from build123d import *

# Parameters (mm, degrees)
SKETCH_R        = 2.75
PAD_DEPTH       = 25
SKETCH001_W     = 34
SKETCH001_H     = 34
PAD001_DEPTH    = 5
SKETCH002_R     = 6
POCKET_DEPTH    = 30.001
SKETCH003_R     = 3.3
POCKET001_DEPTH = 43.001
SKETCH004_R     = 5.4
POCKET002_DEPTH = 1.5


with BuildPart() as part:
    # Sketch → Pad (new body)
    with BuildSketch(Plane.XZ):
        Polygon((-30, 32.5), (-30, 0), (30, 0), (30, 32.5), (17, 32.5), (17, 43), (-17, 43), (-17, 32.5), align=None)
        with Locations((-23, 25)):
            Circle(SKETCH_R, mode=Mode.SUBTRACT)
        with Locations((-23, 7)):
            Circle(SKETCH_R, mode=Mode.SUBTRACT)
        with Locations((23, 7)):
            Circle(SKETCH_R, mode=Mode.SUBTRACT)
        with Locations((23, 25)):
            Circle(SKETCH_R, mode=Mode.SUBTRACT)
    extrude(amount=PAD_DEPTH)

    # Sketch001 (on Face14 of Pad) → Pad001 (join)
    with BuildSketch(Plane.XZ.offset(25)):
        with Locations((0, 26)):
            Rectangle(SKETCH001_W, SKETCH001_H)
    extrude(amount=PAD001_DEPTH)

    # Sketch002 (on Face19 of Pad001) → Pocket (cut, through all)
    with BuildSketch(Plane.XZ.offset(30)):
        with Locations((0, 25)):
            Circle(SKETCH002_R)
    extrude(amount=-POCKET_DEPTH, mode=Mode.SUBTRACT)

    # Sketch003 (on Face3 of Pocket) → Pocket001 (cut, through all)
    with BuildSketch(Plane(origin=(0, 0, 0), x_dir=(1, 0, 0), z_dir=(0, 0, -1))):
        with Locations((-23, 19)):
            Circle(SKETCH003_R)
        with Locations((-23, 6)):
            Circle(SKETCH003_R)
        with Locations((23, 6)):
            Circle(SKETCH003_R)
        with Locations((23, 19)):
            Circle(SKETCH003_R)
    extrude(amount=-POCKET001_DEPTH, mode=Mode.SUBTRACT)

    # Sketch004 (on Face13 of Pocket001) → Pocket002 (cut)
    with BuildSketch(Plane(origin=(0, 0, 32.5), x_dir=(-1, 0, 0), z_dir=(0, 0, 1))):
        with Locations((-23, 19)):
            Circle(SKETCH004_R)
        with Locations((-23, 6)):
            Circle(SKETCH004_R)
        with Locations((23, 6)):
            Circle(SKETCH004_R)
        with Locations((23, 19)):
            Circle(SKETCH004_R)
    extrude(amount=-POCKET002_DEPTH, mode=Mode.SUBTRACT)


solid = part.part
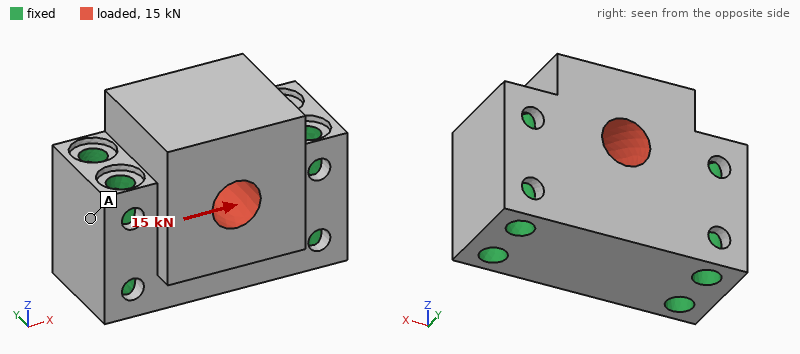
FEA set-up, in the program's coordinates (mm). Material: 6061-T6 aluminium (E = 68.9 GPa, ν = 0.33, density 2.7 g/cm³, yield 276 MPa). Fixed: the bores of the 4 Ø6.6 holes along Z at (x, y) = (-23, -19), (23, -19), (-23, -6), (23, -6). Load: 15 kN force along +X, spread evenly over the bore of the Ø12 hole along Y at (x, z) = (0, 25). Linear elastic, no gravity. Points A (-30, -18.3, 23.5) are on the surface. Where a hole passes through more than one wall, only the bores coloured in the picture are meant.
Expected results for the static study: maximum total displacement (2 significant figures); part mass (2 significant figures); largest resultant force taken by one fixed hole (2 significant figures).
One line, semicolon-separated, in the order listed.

5.5 µm; 150 g; 4.2 kN
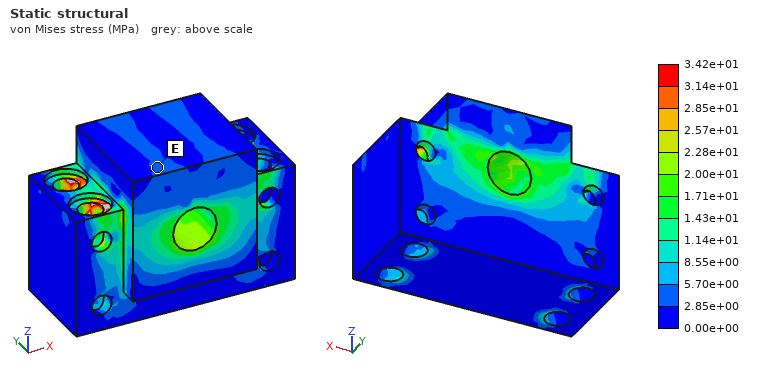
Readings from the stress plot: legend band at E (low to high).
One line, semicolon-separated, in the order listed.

2.85e+00 to 5.70e+00 MPa
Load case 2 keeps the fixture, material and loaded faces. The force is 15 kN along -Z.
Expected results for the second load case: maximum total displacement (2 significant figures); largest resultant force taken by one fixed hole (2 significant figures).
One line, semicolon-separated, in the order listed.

9.7 µm; 4.5 kN
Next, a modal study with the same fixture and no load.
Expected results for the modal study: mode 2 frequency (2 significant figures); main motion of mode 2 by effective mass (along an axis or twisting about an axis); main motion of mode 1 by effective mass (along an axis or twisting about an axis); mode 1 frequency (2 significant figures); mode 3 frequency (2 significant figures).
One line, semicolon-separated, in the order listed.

29 kHz; along Z; along Y; 19 kHz; 31 kHz
